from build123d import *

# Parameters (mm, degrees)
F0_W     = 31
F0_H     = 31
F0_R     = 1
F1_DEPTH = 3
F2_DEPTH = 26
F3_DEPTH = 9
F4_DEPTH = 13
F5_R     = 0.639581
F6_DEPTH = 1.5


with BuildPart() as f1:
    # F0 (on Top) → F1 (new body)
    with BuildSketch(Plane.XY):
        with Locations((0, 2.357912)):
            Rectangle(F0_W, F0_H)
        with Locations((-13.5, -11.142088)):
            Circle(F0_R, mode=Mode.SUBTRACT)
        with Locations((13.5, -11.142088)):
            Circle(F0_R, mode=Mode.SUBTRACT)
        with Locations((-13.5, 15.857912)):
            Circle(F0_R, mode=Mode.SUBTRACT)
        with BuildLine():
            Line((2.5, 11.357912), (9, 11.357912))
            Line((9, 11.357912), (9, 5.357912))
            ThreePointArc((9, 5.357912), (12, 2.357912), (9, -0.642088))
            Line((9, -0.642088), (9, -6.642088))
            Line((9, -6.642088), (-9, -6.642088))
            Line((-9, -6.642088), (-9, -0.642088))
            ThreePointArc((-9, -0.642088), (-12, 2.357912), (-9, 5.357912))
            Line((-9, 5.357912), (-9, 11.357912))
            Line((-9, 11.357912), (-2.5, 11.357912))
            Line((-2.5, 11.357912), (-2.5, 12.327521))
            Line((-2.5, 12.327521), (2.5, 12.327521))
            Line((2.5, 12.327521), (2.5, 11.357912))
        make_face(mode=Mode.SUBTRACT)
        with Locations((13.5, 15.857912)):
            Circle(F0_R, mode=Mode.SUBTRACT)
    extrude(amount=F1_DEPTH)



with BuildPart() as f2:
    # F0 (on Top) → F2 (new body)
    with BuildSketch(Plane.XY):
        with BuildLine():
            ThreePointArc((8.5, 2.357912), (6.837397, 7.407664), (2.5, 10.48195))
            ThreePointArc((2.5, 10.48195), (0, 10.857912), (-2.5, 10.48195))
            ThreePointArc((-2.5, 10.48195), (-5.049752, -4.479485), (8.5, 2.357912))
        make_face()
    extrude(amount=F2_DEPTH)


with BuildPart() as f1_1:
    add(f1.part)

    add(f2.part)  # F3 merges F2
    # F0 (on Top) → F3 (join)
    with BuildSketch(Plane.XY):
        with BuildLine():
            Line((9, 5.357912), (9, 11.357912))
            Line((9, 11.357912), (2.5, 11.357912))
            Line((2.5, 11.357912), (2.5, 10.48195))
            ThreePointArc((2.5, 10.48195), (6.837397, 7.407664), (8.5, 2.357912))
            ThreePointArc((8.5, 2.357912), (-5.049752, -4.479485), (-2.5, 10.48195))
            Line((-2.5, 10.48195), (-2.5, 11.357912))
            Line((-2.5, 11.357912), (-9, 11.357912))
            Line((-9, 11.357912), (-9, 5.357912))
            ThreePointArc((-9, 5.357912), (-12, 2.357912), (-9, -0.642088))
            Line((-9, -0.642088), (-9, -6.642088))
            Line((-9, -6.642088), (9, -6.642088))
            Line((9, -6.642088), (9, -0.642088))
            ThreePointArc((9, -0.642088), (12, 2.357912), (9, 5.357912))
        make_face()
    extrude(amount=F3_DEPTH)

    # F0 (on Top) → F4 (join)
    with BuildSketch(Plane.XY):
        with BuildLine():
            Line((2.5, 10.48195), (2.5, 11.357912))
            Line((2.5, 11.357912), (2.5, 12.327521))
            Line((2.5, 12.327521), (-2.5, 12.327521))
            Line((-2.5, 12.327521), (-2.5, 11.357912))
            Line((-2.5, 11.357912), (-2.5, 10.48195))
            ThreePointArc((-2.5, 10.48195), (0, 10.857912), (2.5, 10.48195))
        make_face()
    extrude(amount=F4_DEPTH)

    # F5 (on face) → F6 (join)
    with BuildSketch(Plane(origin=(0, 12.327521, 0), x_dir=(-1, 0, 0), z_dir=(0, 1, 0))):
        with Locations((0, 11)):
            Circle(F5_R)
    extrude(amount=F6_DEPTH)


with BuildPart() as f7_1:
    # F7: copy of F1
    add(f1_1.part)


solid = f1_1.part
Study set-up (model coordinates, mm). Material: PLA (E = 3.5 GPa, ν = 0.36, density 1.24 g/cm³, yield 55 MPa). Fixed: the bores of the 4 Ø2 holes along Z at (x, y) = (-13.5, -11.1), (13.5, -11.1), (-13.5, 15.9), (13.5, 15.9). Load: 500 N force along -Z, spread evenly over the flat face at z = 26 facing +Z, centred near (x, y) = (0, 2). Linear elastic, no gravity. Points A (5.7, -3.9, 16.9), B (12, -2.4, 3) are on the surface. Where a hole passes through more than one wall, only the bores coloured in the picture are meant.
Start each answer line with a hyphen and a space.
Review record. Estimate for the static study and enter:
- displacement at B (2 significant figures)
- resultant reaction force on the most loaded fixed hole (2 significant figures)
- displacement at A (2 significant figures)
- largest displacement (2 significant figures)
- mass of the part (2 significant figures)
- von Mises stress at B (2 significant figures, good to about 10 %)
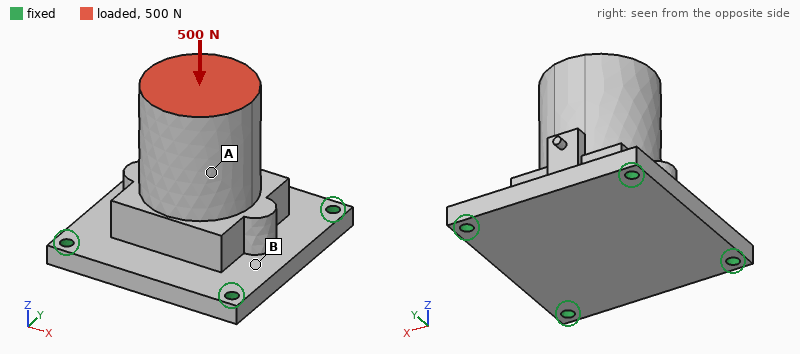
- 0.12 mm
- 130 N
- 0.15 mm
- 0.15 mm
- 11 g
- 11 MPa
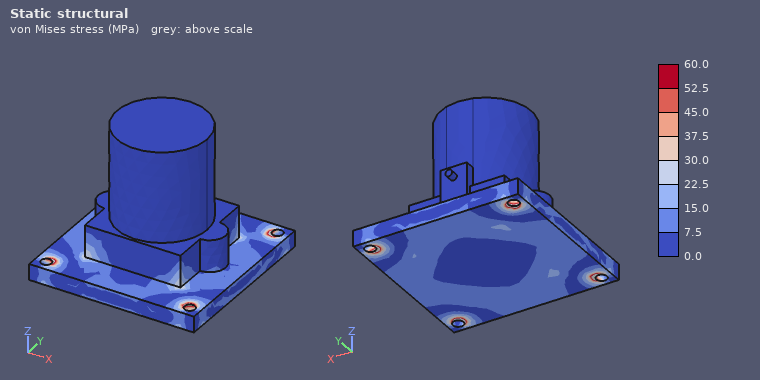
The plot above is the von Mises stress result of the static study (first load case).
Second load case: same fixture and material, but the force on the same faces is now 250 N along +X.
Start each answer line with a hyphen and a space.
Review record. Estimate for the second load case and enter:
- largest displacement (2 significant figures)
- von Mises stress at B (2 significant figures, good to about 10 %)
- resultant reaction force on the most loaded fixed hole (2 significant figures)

- 0.41 mm
- 15 MPa
- 150 N
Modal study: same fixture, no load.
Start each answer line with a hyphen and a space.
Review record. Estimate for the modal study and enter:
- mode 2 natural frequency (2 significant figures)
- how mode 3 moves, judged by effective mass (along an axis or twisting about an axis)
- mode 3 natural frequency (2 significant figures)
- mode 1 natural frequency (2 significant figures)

- 2500 Hz
- along Z
- 3000 Hz
- 2500 Hz
